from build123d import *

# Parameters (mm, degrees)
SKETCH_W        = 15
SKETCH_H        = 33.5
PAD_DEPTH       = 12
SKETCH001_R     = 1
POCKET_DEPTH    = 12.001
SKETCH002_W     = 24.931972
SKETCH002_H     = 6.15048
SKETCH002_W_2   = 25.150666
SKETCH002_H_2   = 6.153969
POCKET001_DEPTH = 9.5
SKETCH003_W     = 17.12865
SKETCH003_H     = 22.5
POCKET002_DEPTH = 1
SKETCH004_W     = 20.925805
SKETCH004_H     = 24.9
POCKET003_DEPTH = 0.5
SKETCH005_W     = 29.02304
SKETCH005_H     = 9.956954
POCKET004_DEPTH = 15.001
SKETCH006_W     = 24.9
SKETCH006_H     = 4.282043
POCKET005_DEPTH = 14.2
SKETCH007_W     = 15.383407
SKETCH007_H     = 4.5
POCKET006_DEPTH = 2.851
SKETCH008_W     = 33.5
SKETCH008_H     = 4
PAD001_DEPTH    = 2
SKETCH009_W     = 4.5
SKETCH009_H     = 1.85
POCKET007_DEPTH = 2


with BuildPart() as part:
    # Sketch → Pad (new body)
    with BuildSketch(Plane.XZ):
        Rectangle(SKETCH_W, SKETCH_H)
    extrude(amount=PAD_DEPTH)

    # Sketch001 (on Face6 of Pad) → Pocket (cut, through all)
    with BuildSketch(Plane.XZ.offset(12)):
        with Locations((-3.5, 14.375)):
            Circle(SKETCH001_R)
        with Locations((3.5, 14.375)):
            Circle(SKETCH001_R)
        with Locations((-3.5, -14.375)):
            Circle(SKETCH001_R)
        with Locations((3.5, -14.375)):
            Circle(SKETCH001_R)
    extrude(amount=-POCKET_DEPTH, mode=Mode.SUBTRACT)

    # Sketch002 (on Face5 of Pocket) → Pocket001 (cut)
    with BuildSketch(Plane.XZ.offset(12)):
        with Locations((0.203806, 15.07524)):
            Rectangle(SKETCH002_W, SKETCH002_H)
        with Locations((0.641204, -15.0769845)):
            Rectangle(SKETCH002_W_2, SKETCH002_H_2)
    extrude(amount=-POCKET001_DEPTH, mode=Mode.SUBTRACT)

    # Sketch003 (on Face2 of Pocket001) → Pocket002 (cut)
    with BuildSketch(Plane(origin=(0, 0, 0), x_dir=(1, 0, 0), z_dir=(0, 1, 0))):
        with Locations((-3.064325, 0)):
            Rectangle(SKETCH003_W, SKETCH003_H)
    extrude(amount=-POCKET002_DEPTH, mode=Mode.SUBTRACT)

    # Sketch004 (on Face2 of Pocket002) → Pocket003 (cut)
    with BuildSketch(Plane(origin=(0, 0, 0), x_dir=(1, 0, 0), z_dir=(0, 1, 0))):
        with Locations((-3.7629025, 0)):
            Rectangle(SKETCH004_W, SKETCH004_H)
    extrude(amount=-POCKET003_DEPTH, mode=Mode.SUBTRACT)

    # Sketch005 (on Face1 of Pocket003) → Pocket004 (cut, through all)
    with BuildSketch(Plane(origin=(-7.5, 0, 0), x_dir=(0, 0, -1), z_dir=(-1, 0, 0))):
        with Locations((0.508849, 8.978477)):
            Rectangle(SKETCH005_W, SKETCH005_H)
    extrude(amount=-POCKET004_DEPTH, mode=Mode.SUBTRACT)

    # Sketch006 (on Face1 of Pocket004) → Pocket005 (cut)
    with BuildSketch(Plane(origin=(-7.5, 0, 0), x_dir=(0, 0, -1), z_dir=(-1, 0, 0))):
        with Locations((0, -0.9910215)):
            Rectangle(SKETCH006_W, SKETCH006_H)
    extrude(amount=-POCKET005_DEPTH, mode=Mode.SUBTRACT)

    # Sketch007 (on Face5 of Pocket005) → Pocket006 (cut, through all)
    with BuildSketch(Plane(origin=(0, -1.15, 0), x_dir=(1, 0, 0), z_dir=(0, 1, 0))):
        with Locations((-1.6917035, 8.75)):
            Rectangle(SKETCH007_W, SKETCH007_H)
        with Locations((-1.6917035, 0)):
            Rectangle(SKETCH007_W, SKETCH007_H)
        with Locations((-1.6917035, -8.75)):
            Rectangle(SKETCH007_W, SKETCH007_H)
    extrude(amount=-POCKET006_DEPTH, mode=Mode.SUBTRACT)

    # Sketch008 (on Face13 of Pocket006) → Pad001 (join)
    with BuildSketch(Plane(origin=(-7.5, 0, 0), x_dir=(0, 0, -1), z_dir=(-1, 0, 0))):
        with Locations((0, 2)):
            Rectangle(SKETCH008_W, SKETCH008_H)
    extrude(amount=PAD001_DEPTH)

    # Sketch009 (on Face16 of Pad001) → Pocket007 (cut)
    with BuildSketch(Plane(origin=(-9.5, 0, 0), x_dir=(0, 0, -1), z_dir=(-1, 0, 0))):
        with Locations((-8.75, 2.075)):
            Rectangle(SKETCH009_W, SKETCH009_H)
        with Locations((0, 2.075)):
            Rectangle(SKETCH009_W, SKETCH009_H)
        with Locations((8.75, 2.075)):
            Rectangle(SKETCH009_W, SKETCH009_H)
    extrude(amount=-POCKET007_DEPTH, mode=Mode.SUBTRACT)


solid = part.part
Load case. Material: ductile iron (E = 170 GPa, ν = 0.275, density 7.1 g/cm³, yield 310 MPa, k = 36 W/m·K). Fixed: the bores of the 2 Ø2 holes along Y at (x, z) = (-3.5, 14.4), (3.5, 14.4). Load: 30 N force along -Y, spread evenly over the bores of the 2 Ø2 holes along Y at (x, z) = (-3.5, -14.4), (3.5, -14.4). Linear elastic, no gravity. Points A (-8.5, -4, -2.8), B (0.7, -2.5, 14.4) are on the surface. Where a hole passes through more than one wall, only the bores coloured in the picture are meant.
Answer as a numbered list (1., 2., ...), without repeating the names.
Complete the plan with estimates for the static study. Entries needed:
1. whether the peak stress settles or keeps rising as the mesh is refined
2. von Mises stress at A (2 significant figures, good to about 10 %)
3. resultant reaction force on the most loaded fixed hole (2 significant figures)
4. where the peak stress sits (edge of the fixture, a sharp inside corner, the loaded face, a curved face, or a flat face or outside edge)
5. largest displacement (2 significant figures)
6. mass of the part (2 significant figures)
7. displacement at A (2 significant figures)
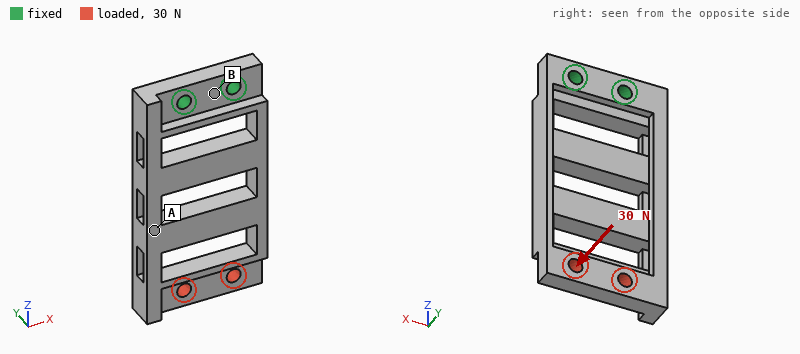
1. keeps rising
2. 34 MPa
3. 20 N
4. a sharp inside corner
5. 0.14 mm
6. 7.5 g
7. 0.062 mm
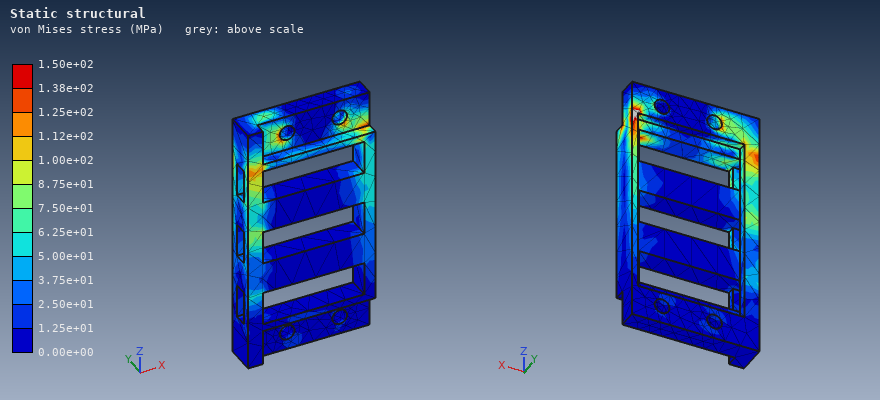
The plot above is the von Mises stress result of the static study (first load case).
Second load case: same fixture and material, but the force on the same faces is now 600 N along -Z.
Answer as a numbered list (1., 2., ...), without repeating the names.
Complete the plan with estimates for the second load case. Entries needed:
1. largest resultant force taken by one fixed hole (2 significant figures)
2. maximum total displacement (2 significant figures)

1. 330 N
2. 92 µm
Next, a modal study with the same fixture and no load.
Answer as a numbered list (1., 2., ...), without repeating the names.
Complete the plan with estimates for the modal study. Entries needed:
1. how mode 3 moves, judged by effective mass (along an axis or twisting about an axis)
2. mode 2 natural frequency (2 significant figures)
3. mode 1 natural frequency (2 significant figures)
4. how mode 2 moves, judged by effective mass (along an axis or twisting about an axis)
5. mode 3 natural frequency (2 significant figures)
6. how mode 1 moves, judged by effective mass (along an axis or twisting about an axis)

1. along X
2. 4200 Hz
3. 1600 Hz
4. along X
5. 5400 Hz
6. along Y
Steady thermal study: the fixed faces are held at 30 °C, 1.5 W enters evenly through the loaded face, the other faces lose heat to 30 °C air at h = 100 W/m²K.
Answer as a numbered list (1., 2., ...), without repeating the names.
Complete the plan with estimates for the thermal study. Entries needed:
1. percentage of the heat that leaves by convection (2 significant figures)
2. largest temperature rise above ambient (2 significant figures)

1. 92 %
2. 27 K
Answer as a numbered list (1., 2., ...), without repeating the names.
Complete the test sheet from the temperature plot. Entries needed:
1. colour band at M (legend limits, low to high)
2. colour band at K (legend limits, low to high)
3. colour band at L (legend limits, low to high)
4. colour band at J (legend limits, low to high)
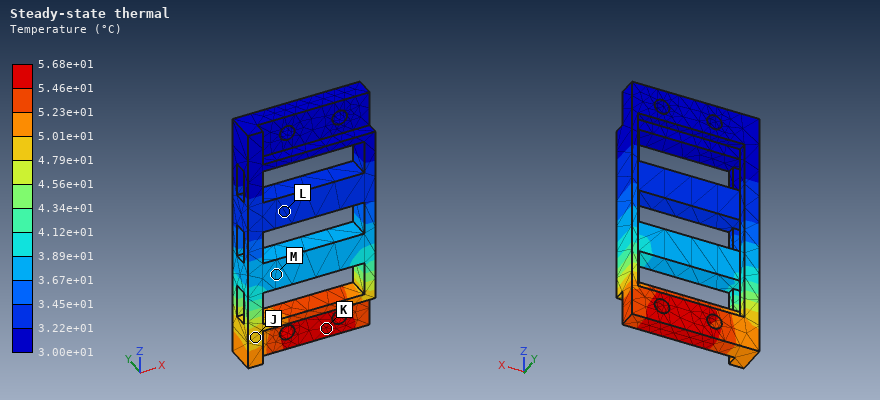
1. 3.67e+01 to 3.89e+01 °C
2. 5.46e+01 to 5.68e+01 °C
3. 3.22e+01 to 3.45e+01 °C
4. 4.79e+01 to 5.01e+01 °C
